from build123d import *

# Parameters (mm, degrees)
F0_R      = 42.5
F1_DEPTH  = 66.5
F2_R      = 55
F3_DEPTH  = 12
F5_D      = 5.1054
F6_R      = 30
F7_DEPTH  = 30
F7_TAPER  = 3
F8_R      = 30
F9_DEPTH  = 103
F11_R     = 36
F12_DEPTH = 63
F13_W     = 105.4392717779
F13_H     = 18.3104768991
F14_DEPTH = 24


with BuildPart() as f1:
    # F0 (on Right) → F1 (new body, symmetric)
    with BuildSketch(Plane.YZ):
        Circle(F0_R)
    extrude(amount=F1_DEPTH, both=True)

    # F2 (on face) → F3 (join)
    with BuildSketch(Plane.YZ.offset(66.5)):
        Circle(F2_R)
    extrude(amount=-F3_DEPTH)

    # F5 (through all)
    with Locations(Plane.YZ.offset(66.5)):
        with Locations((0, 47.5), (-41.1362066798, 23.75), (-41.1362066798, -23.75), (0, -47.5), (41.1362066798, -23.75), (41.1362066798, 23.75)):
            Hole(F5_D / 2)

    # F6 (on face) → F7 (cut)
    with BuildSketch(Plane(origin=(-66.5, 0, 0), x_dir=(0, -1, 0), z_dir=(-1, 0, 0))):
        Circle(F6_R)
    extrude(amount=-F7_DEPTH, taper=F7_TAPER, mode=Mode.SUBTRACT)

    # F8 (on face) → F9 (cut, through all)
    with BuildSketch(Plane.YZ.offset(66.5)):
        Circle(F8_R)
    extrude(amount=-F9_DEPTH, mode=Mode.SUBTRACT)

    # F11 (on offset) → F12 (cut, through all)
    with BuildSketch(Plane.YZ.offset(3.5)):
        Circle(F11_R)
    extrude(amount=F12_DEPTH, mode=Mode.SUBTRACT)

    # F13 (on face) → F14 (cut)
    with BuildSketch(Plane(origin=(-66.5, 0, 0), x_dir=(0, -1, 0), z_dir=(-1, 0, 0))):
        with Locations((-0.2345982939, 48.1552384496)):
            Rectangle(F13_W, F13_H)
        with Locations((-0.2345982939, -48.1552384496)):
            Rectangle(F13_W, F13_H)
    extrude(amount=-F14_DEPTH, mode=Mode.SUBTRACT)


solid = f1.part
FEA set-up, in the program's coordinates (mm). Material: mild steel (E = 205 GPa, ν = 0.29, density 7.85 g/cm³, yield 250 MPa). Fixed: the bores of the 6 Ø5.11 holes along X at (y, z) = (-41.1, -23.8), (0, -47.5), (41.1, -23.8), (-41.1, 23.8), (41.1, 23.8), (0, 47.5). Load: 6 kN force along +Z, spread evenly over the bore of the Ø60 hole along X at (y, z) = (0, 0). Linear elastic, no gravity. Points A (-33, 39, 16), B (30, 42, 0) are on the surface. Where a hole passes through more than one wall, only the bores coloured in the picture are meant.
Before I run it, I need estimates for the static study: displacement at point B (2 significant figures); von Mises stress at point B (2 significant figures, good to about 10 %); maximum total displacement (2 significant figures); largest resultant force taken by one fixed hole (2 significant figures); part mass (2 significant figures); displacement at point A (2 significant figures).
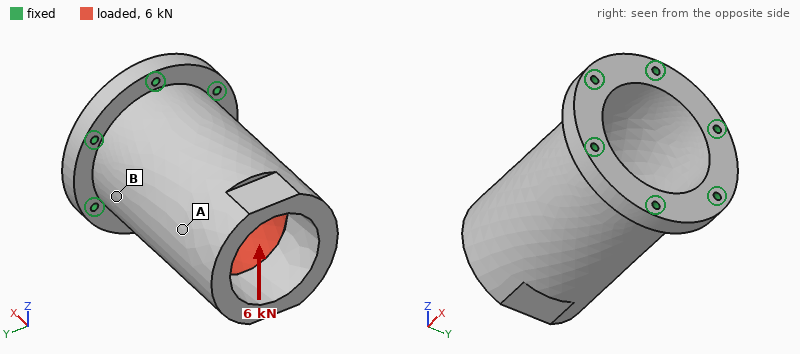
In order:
4.2 µm
11 MPa
19 µm
3.6 kN
2.7 kg
15 µm
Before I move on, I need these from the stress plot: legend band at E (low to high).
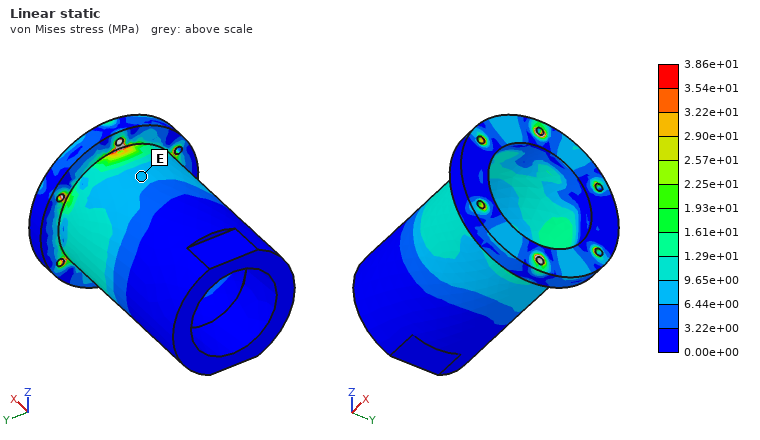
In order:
6.44e+00 to 9.65e+00 MPa
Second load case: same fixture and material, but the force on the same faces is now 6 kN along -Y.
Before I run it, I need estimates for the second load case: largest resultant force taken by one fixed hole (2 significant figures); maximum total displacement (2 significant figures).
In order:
3.1 kN
19 µm
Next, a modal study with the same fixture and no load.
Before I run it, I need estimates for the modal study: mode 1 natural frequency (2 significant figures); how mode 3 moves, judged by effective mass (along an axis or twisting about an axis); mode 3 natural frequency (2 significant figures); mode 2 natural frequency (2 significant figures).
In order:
2200 Hz
twisting about X
5400 Hz
2200 Hz
